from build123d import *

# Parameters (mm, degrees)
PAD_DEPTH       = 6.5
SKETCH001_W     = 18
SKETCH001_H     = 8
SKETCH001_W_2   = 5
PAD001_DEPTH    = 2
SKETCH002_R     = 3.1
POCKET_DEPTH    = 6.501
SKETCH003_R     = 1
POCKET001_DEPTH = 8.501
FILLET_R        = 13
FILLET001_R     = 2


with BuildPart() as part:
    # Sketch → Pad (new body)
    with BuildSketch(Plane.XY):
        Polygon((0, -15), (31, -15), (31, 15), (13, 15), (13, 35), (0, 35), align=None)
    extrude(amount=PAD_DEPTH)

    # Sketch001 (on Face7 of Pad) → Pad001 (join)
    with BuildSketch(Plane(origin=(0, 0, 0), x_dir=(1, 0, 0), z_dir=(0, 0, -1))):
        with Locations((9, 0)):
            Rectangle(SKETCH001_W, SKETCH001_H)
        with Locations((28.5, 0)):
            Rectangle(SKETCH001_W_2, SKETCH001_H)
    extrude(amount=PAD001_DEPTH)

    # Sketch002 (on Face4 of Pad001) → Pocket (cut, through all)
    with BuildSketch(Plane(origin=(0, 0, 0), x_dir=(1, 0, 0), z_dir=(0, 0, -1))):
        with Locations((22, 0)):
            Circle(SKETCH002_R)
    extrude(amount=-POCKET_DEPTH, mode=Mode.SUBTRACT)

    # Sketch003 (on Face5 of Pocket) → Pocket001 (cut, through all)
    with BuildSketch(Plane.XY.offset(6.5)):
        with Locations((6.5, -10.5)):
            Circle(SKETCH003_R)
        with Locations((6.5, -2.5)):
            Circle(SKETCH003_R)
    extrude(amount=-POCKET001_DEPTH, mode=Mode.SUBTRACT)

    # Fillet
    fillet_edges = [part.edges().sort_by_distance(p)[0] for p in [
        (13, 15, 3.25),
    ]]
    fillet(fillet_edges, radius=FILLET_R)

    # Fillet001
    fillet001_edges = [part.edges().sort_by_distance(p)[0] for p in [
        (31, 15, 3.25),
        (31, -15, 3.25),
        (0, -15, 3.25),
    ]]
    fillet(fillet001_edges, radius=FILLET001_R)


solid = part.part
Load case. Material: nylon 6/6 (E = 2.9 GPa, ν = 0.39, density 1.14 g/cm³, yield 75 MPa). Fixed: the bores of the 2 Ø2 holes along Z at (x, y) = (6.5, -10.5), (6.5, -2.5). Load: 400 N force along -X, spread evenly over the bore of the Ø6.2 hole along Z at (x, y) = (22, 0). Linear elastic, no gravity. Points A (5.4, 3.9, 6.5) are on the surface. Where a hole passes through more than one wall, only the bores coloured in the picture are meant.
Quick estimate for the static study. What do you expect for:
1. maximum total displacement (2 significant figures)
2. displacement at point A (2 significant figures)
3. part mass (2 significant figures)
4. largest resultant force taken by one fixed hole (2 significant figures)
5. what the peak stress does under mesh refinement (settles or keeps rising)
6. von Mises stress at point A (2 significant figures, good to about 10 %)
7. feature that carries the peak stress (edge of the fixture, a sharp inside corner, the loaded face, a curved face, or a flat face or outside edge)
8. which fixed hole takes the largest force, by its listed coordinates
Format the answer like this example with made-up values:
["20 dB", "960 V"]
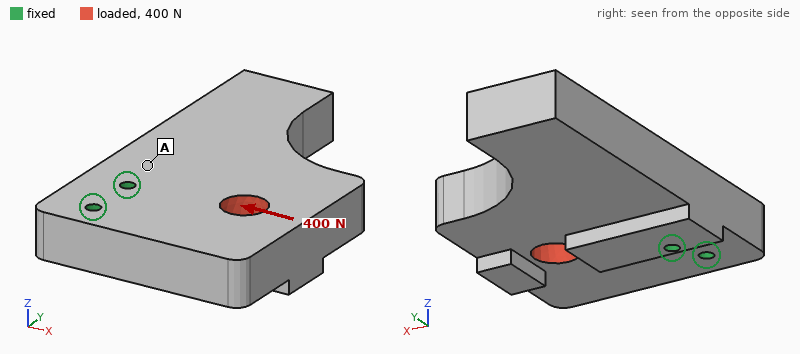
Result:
["0.14 mm", "0.034 mm", "9.2 g", "480 N", "keeps rising", "2.6 MPa", "edge of the fixture", "(6.5, -2.5)"]
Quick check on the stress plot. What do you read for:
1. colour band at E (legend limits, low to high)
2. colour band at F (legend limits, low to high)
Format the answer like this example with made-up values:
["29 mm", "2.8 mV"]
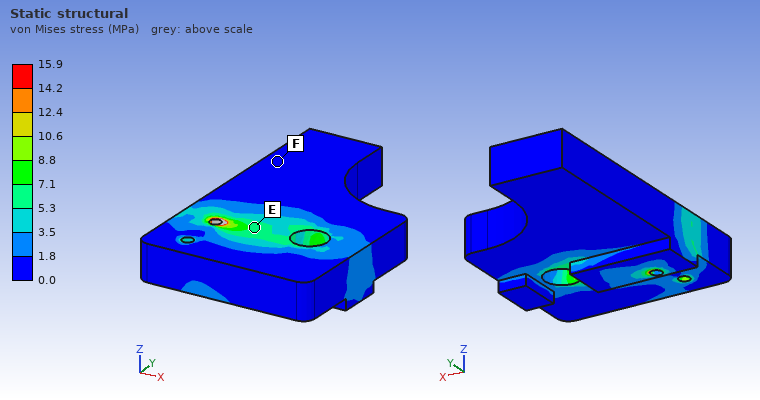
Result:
["5.3 to 7.1 MPa", "0.0 to 1.8 MPa"]
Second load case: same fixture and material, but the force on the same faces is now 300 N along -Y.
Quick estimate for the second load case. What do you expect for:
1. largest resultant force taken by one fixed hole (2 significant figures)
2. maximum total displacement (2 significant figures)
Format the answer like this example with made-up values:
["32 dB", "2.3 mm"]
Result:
["510 N", "0.26 mm"]
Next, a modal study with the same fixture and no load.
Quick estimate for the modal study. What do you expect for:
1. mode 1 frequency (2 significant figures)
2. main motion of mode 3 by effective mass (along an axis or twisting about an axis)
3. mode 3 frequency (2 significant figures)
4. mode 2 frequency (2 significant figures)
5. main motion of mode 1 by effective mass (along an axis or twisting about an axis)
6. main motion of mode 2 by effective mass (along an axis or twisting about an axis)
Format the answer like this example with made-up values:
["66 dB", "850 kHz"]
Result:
["1400 Hz", "along Z", "2400 Hz", "2100 Hz", "along Z", "along X"]
